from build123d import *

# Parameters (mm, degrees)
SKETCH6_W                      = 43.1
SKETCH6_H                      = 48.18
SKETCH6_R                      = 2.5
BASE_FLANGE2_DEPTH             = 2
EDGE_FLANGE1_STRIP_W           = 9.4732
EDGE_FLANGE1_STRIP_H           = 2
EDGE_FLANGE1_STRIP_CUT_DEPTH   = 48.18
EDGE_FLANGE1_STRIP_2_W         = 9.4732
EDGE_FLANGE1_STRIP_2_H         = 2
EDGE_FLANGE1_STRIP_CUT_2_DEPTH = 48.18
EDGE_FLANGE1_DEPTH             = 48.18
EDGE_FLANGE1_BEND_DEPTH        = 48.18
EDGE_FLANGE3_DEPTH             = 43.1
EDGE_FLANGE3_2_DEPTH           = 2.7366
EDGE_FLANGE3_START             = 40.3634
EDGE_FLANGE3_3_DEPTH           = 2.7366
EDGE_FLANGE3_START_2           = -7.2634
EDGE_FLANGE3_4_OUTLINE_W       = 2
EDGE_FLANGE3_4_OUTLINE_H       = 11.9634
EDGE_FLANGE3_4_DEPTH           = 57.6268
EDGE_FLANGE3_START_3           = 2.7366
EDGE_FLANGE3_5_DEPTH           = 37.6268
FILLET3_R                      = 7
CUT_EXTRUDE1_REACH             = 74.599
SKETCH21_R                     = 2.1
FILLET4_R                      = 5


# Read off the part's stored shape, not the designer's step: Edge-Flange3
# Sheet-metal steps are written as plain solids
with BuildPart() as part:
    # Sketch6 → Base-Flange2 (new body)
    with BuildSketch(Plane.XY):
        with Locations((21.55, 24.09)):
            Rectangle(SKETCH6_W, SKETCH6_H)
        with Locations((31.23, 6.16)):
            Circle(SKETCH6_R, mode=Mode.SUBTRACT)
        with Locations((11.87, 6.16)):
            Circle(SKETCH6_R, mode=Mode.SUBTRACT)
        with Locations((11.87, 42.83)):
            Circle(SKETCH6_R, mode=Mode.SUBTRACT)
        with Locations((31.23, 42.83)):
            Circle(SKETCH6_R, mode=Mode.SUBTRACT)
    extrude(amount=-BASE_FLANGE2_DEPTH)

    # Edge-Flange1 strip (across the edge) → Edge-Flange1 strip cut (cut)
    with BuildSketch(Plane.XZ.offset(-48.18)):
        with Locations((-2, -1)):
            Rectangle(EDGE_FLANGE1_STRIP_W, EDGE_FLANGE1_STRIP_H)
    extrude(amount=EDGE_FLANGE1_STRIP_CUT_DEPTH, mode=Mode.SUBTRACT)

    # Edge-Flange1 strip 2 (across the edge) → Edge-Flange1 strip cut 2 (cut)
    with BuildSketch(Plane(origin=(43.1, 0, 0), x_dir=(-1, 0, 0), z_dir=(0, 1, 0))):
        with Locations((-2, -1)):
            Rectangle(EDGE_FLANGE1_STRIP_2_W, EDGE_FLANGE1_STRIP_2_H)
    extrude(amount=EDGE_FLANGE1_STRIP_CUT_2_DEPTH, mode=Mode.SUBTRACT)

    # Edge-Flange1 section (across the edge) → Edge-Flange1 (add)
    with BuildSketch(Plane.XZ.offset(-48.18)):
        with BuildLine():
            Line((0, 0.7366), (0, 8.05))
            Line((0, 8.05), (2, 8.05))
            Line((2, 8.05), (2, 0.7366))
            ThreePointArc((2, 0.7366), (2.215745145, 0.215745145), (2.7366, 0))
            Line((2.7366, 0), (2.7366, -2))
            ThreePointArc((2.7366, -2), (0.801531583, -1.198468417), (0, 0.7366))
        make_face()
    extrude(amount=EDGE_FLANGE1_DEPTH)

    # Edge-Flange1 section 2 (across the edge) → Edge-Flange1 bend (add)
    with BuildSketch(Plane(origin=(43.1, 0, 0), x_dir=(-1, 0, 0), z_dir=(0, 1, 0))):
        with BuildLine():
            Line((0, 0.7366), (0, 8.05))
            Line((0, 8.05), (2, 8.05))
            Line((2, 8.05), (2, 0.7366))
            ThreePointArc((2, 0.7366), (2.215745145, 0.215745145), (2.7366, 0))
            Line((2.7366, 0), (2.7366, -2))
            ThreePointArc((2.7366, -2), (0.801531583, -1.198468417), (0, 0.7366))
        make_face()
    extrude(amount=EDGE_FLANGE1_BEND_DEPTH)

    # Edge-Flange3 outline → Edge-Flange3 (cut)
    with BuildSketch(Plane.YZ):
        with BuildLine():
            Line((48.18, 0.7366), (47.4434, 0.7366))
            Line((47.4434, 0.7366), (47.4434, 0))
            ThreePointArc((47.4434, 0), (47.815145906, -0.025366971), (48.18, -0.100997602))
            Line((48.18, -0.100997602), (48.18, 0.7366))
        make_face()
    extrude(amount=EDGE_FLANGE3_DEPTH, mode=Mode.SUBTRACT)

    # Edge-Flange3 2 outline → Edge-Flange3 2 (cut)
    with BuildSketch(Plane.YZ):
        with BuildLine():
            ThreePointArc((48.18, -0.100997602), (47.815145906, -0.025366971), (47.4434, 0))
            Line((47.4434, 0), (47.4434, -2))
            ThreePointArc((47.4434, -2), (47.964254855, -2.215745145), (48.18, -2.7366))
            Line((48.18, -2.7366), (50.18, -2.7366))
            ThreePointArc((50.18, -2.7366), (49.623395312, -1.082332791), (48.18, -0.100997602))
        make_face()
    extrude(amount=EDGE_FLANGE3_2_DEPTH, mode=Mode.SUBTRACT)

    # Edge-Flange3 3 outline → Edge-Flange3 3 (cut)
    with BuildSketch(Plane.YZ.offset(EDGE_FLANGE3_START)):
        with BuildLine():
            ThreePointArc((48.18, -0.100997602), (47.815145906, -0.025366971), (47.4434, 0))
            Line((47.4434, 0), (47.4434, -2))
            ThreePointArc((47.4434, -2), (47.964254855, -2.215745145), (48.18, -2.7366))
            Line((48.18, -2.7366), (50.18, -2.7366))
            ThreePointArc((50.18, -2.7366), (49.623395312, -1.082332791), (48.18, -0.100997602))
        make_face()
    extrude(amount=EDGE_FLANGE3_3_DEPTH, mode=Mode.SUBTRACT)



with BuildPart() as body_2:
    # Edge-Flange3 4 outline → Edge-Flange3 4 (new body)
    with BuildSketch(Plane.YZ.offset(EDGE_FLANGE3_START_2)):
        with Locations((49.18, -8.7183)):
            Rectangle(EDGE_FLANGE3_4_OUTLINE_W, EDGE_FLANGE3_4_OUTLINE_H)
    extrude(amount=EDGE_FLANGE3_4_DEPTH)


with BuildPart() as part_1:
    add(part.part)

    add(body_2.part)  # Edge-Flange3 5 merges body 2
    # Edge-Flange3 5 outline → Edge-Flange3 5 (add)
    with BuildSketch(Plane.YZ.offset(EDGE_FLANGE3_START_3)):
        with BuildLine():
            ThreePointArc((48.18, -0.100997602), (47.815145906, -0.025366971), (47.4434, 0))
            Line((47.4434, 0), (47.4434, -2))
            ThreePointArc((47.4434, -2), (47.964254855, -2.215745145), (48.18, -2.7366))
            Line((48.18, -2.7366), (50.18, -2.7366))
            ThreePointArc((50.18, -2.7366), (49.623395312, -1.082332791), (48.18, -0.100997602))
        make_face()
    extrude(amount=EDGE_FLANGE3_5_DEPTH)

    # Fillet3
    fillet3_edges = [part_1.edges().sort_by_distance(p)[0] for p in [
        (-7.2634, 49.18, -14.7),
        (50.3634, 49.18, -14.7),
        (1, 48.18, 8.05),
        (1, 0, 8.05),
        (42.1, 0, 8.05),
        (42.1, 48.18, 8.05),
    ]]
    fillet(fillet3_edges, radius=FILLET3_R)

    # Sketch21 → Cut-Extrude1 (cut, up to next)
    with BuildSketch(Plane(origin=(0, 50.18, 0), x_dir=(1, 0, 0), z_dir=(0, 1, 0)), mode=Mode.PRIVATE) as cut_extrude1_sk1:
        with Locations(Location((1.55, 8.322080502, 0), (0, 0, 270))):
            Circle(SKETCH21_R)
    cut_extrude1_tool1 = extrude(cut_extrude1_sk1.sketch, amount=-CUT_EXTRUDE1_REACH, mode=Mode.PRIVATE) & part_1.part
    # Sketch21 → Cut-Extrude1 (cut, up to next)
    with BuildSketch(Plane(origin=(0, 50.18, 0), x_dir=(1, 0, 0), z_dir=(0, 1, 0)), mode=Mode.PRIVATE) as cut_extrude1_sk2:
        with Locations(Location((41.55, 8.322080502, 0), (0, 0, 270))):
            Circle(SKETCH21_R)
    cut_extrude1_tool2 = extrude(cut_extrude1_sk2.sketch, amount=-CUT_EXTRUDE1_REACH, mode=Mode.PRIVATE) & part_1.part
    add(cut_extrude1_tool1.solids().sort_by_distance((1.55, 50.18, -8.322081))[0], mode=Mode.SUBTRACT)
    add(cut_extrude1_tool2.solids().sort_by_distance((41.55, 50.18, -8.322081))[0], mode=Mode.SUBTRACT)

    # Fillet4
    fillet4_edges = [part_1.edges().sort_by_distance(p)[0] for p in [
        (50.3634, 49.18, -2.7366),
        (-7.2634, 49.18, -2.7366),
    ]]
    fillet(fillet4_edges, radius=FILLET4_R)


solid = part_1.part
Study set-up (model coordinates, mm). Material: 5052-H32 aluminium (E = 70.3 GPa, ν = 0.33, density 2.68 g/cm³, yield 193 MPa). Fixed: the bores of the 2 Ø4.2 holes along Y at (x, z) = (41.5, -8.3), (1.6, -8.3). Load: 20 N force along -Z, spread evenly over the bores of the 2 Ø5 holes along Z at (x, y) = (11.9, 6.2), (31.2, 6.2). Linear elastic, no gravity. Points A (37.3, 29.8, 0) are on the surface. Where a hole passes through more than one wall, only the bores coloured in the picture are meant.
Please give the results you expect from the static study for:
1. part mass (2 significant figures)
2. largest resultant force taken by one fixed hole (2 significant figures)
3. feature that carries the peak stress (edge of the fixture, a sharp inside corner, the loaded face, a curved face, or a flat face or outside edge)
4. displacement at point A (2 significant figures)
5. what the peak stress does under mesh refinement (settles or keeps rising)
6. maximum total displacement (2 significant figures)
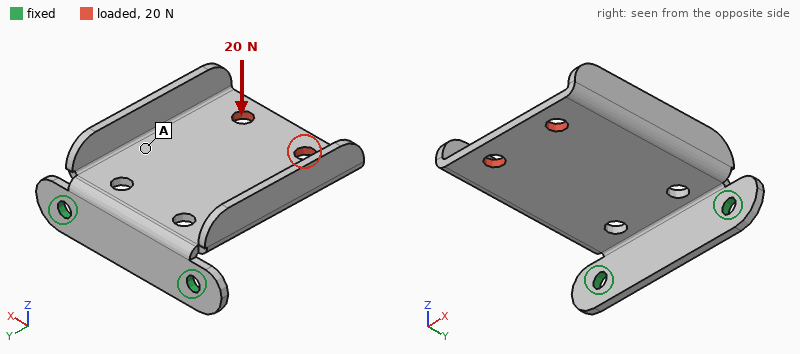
18 g
14 N
a sharp inside corner
0.13 mm
keeps rising
0.37 mm
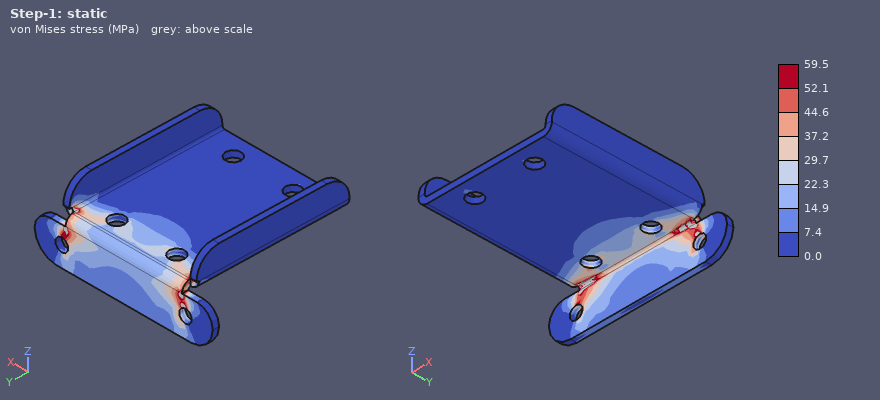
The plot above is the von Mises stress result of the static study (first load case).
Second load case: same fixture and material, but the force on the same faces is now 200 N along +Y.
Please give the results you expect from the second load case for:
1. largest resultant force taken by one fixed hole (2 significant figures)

100 N
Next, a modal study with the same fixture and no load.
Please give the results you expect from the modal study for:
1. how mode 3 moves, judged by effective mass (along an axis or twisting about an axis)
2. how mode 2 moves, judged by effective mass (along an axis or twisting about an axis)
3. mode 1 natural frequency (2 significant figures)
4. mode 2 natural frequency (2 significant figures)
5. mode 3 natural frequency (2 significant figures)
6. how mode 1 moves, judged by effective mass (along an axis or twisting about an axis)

along X
twisting about Y
510 Hz
1300 Hz
2800 Hz
along Z
